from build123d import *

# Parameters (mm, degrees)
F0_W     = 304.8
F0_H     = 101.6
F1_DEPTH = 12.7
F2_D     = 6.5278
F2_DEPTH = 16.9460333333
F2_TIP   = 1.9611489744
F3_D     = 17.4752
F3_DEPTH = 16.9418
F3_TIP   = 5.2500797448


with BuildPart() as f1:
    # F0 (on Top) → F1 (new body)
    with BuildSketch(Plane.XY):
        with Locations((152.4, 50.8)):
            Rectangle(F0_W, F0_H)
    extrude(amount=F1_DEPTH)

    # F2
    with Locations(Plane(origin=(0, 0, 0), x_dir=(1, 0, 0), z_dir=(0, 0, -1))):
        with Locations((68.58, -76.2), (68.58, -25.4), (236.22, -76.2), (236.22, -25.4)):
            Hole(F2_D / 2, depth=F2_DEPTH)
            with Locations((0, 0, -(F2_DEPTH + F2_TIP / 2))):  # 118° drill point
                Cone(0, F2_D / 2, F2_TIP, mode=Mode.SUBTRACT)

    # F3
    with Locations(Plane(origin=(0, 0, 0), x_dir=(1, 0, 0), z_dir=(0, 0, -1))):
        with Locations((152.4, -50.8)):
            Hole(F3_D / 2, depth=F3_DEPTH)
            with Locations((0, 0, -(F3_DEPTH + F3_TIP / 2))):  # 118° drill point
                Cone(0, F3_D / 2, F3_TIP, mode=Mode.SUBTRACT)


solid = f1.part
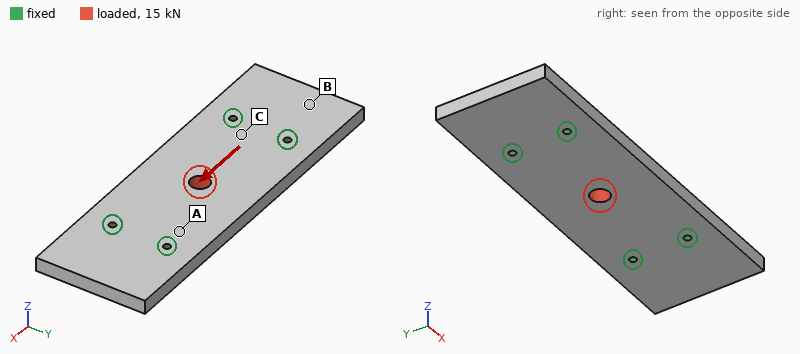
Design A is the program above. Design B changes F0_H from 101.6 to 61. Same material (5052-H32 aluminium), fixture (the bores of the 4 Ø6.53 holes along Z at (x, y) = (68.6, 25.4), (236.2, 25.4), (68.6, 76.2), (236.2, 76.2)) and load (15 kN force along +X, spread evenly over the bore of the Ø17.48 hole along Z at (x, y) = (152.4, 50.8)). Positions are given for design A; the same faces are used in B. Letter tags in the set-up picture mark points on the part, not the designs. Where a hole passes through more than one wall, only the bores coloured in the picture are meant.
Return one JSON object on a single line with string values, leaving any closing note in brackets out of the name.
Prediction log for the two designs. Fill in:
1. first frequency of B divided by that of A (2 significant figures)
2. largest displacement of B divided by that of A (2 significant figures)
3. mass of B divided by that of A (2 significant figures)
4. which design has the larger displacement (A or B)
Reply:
{"first frequency of B divided by that of A": "1.1", "largest displacement of B divided by that of A": "1.2", "mass of B divided by that of A": "0.60", "which design has the larger displacement": "B"}
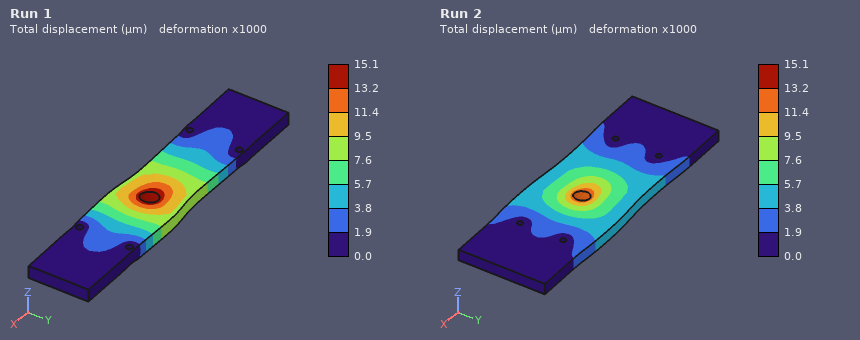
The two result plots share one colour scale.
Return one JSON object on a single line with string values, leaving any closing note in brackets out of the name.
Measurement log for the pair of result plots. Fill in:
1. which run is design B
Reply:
{"which run is design B": "Run 1"}
